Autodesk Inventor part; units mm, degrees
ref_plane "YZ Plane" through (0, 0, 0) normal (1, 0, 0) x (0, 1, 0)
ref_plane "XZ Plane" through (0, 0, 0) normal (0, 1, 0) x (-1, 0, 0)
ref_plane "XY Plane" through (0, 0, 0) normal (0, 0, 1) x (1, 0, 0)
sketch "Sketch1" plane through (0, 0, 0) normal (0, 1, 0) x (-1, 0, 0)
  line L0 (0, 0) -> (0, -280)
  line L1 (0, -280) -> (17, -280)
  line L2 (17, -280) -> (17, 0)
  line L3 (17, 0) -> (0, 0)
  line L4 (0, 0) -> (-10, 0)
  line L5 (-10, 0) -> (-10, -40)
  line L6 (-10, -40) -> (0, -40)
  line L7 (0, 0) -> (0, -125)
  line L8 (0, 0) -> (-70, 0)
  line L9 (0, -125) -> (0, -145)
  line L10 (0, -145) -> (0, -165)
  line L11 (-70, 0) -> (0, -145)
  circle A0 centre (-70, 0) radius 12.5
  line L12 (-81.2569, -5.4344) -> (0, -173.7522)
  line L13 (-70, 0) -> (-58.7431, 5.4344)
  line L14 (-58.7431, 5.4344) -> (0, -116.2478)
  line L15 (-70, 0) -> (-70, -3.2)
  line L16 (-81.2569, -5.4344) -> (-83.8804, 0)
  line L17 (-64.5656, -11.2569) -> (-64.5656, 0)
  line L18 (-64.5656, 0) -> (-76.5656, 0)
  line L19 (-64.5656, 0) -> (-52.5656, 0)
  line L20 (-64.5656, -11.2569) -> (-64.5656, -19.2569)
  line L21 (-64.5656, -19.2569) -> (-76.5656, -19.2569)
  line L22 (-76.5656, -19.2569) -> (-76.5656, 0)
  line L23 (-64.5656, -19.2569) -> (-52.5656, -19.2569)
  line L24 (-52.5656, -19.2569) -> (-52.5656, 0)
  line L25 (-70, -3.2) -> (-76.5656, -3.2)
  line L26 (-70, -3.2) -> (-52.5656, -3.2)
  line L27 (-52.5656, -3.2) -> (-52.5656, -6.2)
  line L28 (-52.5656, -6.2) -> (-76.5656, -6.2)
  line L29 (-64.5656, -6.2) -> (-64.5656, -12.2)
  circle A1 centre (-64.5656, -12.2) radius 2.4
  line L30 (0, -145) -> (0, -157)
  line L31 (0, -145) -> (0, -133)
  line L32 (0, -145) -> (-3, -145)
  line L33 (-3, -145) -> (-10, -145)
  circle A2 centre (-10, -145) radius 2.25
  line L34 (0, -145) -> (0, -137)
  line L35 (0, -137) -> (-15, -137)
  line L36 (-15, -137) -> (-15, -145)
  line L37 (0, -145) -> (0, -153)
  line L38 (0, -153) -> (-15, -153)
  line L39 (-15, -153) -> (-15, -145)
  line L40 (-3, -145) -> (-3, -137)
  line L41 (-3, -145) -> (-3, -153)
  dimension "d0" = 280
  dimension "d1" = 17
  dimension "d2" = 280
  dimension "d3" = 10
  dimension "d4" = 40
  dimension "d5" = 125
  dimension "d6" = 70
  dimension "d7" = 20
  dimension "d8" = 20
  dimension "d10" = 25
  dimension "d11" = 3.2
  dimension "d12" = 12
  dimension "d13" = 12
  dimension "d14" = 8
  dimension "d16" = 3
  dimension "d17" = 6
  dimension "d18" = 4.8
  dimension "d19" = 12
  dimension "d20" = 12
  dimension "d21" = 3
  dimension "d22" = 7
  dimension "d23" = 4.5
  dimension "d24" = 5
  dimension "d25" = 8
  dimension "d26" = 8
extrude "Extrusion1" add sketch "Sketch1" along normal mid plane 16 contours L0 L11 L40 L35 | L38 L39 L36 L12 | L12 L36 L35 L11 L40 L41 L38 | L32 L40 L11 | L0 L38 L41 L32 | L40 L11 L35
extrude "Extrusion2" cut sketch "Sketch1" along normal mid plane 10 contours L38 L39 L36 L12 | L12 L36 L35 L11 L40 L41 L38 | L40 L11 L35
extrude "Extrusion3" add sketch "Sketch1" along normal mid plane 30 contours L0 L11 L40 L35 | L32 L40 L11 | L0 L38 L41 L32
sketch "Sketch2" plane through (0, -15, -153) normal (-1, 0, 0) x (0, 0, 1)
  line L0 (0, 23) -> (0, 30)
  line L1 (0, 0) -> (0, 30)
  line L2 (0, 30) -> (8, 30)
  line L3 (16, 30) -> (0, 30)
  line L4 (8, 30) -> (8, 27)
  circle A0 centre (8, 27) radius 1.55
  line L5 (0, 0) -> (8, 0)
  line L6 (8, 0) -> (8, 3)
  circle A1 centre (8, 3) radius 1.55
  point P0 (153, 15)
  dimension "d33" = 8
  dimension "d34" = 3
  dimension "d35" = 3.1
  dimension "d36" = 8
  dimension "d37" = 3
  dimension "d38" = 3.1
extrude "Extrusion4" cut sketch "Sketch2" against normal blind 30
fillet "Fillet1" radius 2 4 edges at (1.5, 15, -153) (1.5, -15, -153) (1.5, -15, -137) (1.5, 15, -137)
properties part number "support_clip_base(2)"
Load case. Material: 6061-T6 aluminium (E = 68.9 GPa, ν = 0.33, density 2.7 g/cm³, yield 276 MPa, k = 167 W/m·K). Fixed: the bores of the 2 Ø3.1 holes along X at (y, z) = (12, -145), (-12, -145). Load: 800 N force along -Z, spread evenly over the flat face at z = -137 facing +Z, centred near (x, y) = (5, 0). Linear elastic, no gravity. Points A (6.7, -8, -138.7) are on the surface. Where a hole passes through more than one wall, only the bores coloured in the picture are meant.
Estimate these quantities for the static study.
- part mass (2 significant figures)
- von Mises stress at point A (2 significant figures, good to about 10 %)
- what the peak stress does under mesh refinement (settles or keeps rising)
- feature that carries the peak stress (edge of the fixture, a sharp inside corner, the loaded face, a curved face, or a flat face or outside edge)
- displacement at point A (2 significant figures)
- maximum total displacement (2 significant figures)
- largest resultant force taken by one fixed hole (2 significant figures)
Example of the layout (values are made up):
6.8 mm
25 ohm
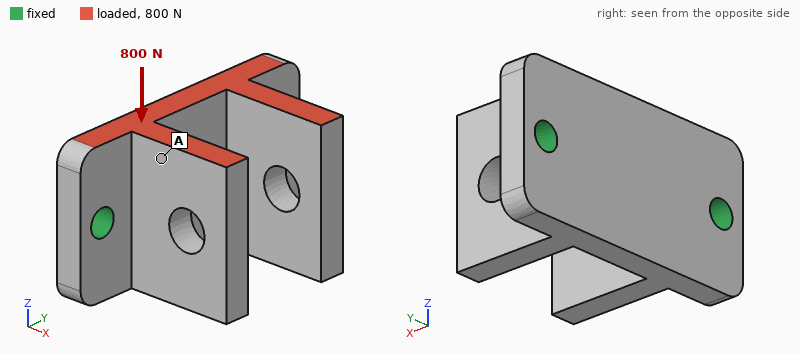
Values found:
6.6 g
14 MPa
keeps rising
edge of the fixture
18 µm
34 µm
400 N
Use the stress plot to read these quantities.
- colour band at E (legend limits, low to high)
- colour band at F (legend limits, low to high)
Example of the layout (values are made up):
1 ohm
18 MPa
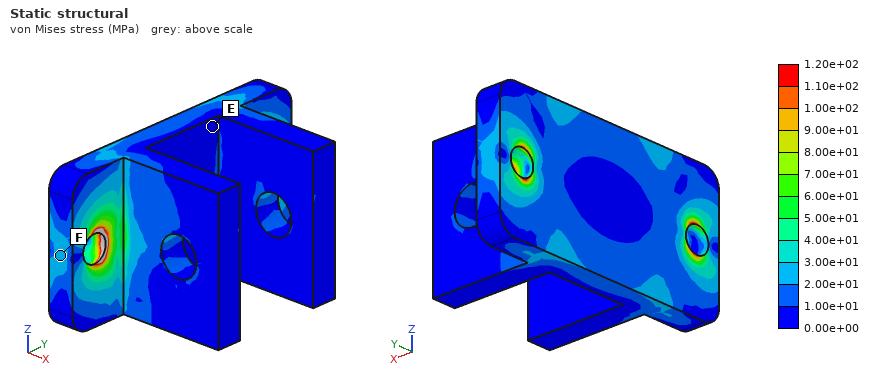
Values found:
0.00e+00 to 1.00e+01 MPa
2.00e+01 to 3.00e+01 MPa
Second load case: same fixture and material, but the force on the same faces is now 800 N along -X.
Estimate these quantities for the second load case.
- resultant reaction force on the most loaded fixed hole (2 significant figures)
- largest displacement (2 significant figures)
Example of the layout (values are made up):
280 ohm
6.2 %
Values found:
400 N
75 µm
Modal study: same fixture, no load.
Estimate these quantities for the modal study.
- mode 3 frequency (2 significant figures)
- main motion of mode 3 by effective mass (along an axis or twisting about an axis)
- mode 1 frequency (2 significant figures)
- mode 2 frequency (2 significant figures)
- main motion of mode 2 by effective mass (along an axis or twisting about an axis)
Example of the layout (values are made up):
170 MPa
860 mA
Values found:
13 kHz
along Y
10 kHz
11 kHz
along Z
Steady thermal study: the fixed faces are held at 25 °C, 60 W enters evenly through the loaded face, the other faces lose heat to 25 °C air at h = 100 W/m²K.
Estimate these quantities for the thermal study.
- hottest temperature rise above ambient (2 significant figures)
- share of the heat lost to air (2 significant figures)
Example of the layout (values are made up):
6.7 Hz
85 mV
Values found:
46 K
7.1 %
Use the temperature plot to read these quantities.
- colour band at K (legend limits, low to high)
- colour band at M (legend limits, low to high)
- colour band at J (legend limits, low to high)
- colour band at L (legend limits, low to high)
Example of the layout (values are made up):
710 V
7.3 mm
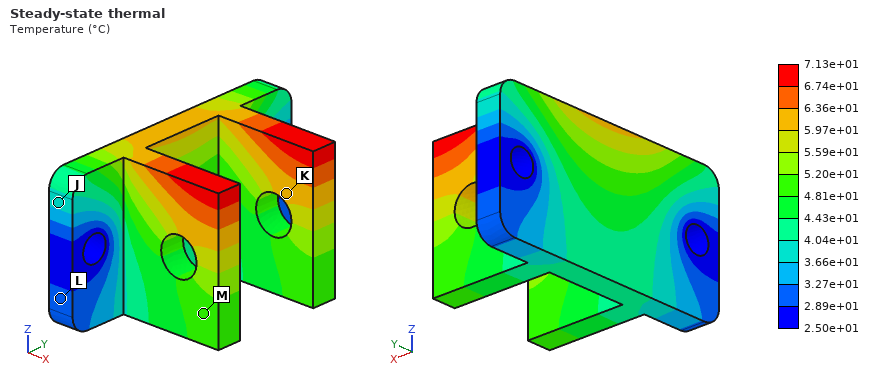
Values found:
5.97e+01 to 6.36e+01 °C
4.81e+01 to 5.20e+01 °C
3.66e+01 to 4.04e+01 °C
2.89e+01 to 3.27e+01 °C
